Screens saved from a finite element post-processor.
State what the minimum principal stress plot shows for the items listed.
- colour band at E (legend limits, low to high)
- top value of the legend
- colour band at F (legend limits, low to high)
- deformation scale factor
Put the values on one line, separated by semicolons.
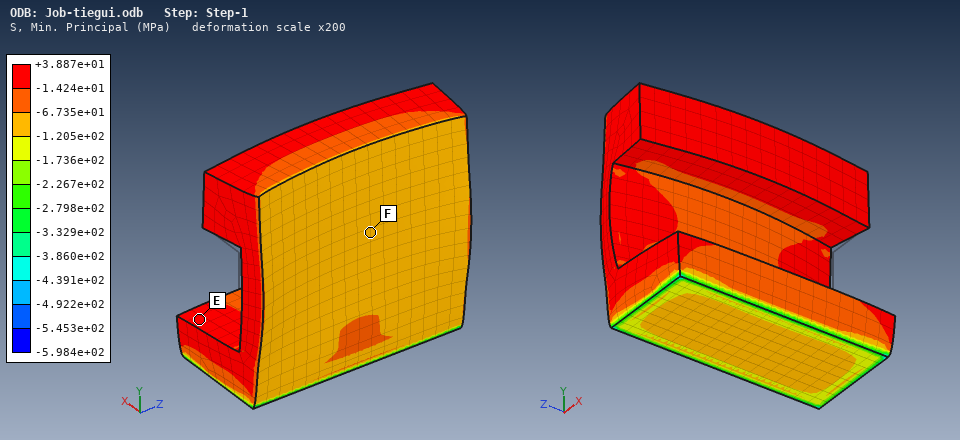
-1.424e+01 to +3.887e+01 MPa; +3.887e+01 MPa; -1.205e+02 to -6.735e+01 MPa; 200
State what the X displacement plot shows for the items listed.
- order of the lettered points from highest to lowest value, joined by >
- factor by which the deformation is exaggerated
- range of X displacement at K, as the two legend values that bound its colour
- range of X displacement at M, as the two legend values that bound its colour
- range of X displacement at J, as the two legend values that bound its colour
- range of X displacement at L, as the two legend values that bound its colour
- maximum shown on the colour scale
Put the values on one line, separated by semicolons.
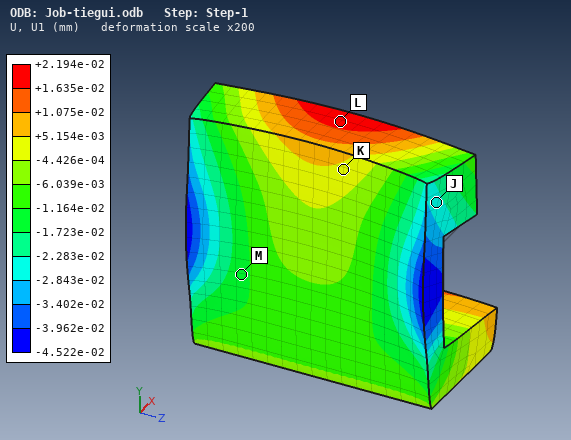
L > K > M > J; 200; -4.426e-04 to +5.154e-03 mm; -1.723e-02 to -1.164e-02 mm; -2.843e-02 to -2.283e-02 mm; +1.635e-02 to +2.194e-02 mm; +2.194e-02 mm
